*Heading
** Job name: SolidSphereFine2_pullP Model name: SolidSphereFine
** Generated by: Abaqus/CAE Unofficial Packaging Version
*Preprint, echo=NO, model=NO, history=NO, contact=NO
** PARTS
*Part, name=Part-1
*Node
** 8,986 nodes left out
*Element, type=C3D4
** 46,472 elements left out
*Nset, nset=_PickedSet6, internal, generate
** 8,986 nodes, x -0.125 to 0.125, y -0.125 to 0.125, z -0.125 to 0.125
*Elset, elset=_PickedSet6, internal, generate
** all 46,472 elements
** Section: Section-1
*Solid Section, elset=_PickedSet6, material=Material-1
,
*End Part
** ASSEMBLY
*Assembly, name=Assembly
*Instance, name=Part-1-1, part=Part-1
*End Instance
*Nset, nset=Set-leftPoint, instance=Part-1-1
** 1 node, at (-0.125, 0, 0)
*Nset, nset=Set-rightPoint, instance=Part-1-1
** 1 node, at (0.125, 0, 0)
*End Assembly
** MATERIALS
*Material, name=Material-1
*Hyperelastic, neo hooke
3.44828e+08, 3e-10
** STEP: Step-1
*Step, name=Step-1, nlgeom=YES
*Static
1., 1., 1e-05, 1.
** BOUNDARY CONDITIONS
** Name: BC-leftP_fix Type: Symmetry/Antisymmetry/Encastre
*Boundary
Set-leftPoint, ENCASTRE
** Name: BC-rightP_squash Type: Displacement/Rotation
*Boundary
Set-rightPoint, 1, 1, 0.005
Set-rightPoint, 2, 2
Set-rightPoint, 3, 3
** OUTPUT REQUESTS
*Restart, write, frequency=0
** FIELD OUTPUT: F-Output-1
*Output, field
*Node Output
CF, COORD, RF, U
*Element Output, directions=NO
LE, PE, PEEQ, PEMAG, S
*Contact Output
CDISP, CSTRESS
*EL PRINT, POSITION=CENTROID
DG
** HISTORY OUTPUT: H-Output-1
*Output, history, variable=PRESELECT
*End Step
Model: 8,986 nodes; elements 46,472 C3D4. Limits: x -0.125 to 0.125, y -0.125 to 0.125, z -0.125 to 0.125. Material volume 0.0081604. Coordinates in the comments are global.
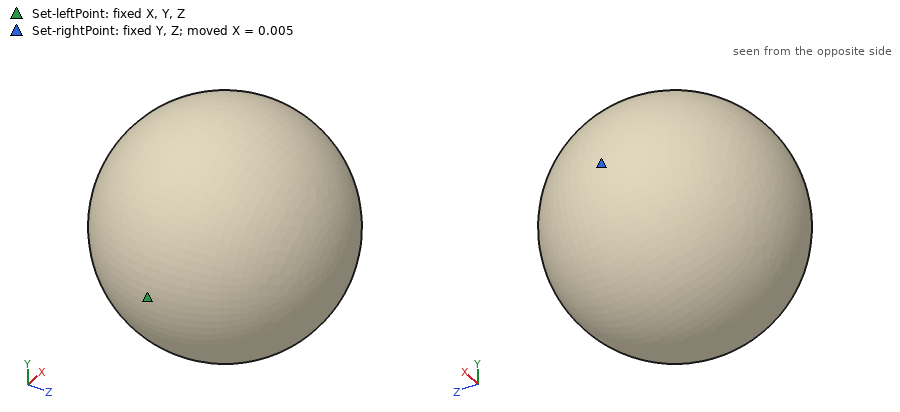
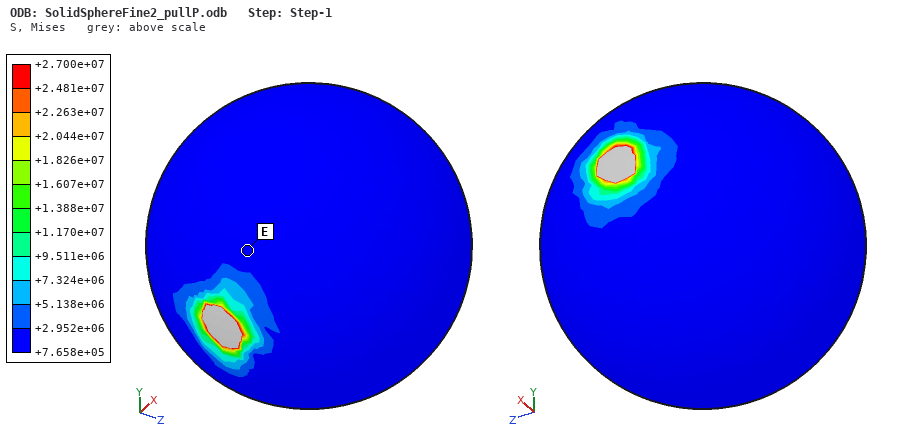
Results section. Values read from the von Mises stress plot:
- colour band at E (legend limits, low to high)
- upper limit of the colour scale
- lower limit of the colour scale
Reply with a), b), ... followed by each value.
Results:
a) +7.658e+05 to +2.952e+06
b) +2.700e+07
c) +7.658e+05
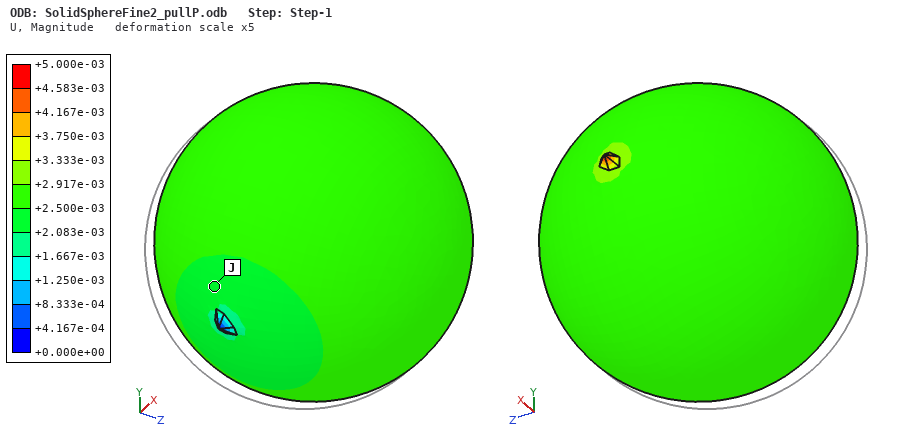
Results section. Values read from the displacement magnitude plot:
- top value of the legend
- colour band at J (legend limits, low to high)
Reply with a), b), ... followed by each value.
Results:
a) +5.000e-03
b) +2.083e-03 to +2.500e-03
